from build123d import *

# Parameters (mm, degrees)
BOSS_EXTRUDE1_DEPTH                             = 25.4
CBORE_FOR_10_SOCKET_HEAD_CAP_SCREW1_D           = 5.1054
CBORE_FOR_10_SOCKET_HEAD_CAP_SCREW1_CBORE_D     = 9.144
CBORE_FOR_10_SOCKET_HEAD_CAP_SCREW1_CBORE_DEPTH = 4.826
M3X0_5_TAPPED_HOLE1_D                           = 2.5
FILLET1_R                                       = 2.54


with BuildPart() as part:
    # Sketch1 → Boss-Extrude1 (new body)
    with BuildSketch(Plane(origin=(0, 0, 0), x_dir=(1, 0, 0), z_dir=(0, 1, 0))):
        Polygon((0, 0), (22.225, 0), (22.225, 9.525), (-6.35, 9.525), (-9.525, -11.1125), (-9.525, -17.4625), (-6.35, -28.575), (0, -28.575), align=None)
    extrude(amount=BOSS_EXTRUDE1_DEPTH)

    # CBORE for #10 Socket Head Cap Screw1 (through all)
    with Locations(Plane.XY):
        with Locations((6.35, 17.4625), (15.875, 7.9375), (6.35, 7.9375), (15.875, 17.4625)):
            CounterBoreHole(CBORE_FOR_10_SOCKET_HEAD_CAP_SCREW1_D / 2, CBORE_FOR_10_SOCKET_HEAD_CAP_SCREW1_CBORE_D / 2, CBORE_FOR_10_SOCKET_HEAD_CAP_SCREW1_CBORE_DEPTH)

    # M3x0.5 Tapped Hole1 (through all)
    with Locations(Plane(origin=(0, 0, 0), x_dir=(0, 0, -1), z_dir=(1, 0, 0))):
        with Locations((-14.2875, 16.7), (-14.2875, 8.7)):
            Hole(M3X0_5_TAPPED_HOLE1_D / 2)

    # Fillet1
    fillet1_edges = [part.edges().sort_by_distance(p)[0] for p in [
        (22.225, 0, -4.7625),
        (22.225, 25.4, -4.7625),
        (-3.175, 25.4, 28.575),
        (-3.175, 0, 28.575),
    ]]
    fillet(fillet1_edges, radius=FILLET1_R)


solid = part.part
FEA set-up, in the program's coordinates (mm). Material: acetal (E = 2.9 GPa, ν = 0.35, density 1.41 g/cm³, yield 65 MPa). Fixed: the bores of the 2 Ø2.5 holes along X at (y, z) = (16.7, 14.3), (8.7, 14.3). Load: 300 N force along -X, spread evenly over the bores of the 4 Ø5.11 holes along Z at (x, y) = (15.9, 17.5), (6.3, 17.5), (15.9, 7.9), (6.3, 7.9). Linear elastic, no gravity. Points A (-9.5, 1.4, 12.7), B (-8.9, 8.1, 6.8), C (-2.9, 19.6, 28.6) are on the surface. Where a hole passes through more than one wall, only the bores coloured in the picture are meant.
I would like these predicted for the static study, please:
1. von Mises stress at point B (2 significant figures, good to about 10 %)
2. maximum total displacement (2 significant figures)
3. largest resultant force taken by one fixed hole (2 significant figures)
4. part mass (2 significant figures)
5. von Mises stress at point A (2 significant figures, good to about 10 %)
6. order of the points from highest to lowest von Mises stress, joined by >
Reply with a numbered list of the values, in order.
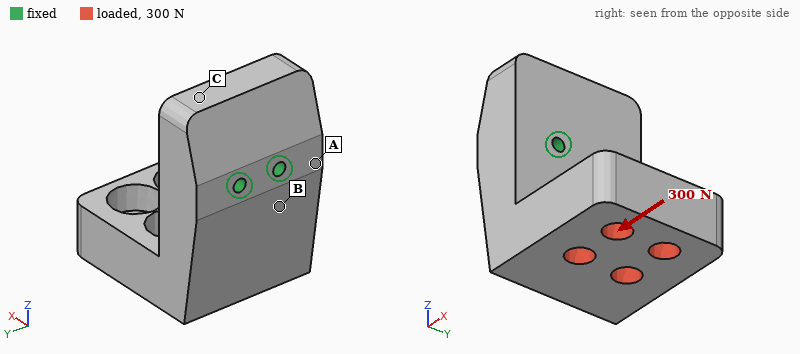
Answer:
1. 13 MPa
2. 0.62 mm
3. 150 N
4. 16 g
5. 7.7 MPa
6. B > A > C
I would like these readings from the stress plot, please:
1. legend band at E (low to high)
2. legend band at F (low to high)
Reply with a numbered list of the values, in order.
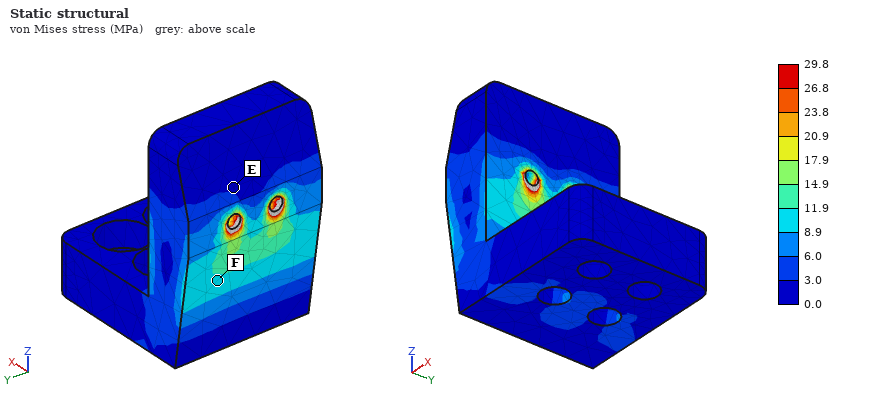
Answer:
1. 0.0 to 3.0 MPa
2. 8.9 to 11.9 MPa
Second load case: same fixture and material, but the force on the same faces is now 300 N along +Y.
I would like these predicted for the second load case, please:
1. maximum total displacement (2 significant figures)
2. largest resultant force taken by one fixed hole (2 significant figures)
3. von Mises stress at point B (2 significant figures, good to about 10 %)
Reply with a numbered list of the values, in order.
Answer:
1. 0.55 mm
2. 710 N
3. 8.3 MPa
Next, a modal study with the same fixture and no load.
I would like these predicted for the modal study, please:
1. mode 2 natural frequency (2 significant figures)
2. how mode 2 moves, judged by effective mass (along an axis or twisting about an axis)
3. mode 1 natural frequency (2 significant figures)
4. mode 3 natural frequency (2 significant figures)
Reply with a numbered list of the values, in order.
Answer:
1. 1800 Hz
2. along Y
3. 1400 Hz
4. 3200 Hz
